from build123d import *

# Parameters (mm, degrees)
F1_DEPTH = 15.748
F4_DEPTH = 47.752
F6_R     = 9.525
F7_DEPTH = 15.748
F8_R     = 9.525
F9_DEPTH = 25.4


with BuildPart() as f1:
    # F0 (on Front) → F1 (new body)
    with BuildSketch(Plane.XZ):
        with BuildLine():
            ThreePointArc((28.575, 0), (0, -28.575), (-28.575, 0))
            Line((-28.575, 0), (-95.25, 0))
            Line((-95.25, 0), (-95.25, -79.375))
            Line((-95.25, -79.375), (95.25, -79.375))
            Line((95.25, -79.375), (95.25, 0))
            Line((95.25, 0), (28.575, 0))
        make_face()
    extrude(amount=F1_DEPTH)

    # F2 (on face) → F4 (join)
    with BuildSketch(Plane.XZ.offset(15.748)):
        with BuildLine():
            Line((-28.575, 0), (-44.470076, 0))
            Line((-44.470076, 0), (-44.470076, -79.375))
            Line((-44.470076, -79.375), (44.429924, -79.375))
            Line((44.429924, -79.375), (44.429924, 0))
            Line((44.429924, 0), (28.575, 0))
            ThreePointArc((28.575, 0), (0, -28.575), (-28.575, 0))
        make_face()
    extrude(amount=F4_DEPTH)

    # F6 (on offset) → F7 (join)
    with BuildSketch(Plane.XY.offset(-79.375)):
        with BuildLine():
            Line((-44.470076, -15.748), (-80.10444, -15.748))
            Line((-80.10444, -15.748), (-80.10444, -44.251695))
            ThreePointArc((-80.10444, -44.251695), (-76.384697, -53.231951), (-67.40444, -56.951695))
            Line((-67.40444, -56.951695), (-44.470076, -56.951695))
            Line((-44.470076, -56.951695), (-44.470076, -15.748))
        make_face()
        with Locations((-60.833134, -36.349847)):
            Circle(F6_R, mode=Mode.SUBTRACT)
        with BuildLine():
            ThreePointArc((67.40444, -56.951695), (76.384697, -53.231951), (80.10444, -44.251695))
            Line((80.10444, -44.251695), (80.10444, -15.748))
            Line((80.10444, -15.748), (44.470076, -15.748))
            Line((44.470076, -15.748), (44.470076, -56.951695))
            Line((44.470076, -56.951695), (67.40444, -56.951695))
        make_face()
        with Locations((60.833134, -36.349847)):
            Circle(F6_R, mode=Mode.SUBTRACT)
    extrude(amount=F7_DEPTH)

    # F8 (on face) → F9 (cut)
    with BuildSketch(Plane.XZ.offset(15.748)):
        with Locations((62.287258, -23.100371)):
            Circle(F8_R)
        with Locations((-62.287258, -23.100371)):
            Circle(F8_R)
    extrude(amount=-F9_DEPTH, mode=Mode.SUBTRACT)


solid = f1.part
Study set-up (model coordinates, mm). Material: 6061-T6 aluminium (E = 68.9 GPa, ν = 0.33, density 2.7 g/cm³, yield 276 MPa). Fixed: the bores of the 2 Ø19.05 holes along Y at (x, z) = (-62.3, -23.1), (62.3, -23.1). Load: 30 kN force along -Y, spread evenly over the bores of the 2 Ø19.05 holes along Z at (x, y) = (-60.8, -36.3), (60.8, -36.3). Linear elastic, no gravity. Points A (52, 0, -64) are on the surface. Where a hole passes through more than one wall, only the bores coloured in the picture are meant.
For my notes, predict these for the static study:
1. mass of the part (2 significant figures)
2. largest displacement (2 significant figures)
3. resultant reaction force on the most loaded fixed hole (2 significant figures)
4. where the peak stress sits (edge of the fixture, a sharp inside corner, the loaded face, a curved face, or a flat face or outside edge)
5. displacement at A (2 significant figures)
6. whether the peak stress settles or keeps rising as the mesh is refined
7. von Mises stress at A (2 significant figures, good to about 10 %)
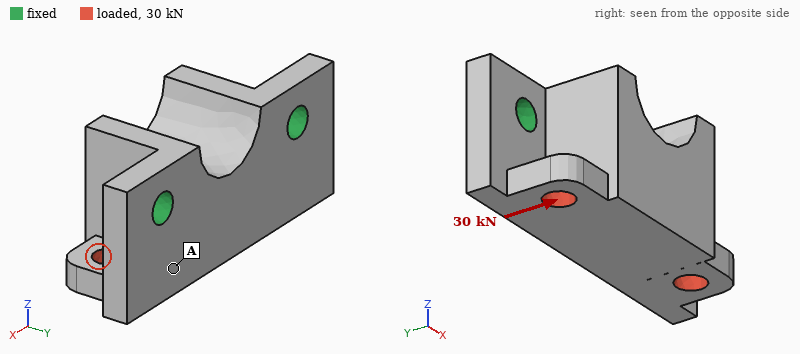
1.4 kg
0.43 mm
15 kN
a sharp inside corner
0.18 mm
keeps rising
45 MPa
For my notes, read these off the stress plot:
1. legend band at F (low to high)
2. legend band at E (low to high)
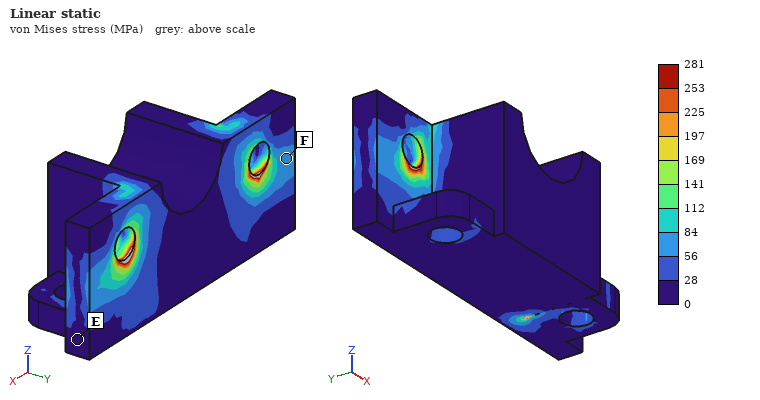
56 to 84 MPa
0 to 28 MPa
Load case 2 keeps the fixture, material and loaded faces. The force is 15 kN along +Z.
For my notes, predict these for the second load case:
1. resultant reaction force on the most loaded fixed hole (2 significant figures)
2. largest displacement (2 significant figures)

7.7 kN
0.37 mm
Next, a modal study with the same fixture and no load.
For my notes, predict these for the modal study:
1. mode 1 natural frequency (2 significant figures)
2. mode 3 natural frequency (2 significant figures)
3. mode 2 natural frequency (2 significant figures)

1800 Hz
5000 Hz
3800 Hz
